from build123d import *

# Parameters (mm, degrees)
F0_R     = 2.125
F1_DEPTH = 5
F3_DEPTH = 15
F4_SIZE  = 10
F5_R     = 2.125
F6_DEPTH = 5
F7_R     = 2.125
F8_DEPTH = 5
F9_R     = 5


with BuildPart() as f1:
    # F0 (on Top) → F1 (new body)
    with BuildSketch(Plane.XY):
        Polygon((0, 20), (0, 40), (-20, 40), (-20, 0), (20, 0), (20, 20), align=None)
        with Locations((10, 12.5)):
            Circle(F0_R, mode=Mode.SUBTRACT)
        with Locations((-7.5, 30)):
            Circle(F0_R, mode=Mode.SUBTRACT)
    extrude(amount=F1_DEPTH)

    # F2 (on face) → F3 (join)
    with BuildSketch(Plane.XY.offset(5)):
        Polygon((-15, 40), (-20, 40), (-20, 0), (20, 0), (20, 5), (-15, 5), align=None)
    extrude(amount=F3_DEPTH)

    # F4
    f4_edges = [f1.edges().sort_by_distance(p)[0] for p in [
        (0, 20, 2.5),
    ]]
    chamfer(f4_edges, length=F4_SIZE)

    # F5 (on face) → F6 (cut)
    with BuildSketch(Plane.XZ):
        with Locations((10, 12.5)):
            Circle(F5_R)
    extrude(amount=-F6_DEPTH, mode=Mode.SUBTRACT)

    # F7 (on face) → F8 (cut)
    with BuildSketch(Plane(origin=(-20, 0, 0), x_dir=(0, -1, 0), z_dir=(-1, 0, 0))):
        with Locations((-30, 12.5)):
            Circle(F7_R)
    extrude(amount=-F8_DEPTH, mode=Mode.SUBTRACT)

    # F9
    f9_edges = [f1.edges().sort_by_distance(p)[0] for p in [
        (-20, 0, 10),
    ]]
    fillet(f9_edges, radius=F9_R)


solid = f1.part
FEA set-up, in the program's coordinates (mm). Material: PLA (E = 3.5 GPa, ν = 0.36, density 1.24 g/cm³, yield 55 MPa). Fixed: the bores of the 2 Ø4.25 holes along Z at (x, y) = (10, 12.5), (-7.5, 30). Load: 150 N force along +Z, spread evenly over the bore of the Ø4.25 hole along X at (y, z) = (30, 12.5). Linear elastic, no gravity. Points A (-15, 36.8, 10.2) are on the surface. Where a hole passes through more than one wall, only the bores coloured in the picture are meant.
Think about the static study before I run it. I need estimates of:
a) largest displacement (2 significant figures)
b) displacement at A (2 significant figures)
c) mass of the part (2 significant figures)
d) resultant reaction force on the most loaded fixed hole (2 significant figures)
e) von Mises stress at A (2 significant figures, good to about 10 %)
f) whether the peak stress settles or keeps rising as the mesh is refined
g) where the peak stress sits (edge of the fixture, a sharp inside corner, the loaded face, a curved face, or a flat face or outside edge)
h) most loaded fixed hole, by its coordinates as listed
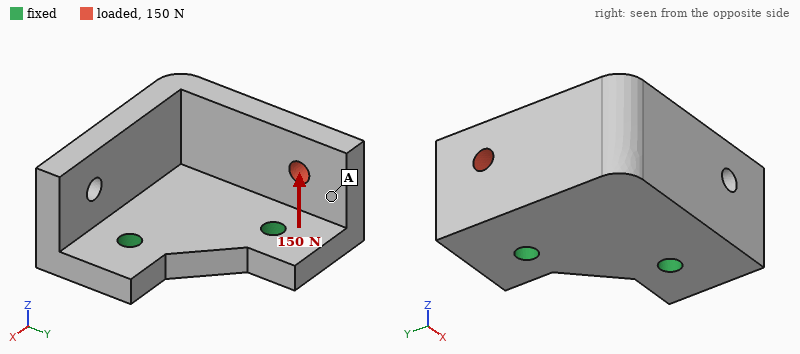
0.15 mm
0.074 mm
14 g
160 N
2.2 MPa
keeps rising
edge of the fixture
(-7.5, 30)
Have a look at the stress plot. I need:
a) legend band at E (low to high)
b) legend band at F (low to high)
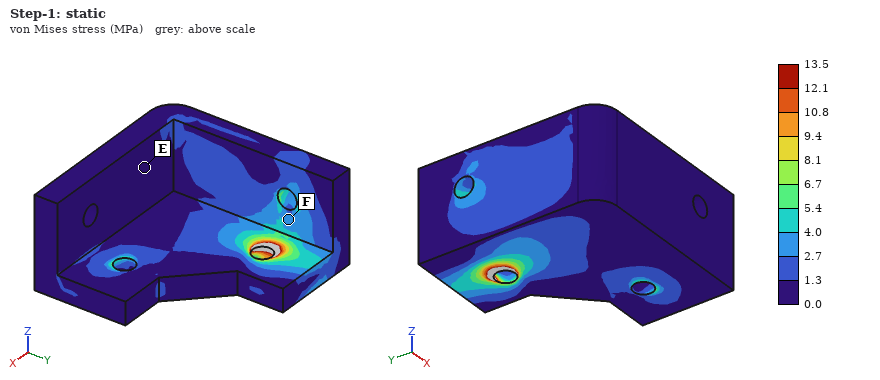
0.0 to 1.3 MPa
2.7 to 4.0 MPa
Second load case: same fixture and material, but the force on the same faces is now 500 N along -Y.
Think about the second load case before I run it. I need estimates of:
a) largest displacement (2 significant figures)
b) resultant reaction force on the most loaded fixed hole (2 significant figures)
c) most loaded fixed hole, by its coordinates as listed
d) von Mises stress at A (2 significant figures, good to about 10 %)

0.64 mm
560 N
(-7.5, 30)
11 MPa
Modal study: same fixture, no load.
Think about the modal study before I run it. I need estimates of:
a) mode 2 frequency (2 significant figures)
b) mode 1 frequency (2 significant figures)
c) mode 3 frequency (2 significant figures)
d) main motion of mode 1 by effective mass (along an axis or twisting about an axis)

2600 Hz
1500 Hz
3500 Hz
along Z
